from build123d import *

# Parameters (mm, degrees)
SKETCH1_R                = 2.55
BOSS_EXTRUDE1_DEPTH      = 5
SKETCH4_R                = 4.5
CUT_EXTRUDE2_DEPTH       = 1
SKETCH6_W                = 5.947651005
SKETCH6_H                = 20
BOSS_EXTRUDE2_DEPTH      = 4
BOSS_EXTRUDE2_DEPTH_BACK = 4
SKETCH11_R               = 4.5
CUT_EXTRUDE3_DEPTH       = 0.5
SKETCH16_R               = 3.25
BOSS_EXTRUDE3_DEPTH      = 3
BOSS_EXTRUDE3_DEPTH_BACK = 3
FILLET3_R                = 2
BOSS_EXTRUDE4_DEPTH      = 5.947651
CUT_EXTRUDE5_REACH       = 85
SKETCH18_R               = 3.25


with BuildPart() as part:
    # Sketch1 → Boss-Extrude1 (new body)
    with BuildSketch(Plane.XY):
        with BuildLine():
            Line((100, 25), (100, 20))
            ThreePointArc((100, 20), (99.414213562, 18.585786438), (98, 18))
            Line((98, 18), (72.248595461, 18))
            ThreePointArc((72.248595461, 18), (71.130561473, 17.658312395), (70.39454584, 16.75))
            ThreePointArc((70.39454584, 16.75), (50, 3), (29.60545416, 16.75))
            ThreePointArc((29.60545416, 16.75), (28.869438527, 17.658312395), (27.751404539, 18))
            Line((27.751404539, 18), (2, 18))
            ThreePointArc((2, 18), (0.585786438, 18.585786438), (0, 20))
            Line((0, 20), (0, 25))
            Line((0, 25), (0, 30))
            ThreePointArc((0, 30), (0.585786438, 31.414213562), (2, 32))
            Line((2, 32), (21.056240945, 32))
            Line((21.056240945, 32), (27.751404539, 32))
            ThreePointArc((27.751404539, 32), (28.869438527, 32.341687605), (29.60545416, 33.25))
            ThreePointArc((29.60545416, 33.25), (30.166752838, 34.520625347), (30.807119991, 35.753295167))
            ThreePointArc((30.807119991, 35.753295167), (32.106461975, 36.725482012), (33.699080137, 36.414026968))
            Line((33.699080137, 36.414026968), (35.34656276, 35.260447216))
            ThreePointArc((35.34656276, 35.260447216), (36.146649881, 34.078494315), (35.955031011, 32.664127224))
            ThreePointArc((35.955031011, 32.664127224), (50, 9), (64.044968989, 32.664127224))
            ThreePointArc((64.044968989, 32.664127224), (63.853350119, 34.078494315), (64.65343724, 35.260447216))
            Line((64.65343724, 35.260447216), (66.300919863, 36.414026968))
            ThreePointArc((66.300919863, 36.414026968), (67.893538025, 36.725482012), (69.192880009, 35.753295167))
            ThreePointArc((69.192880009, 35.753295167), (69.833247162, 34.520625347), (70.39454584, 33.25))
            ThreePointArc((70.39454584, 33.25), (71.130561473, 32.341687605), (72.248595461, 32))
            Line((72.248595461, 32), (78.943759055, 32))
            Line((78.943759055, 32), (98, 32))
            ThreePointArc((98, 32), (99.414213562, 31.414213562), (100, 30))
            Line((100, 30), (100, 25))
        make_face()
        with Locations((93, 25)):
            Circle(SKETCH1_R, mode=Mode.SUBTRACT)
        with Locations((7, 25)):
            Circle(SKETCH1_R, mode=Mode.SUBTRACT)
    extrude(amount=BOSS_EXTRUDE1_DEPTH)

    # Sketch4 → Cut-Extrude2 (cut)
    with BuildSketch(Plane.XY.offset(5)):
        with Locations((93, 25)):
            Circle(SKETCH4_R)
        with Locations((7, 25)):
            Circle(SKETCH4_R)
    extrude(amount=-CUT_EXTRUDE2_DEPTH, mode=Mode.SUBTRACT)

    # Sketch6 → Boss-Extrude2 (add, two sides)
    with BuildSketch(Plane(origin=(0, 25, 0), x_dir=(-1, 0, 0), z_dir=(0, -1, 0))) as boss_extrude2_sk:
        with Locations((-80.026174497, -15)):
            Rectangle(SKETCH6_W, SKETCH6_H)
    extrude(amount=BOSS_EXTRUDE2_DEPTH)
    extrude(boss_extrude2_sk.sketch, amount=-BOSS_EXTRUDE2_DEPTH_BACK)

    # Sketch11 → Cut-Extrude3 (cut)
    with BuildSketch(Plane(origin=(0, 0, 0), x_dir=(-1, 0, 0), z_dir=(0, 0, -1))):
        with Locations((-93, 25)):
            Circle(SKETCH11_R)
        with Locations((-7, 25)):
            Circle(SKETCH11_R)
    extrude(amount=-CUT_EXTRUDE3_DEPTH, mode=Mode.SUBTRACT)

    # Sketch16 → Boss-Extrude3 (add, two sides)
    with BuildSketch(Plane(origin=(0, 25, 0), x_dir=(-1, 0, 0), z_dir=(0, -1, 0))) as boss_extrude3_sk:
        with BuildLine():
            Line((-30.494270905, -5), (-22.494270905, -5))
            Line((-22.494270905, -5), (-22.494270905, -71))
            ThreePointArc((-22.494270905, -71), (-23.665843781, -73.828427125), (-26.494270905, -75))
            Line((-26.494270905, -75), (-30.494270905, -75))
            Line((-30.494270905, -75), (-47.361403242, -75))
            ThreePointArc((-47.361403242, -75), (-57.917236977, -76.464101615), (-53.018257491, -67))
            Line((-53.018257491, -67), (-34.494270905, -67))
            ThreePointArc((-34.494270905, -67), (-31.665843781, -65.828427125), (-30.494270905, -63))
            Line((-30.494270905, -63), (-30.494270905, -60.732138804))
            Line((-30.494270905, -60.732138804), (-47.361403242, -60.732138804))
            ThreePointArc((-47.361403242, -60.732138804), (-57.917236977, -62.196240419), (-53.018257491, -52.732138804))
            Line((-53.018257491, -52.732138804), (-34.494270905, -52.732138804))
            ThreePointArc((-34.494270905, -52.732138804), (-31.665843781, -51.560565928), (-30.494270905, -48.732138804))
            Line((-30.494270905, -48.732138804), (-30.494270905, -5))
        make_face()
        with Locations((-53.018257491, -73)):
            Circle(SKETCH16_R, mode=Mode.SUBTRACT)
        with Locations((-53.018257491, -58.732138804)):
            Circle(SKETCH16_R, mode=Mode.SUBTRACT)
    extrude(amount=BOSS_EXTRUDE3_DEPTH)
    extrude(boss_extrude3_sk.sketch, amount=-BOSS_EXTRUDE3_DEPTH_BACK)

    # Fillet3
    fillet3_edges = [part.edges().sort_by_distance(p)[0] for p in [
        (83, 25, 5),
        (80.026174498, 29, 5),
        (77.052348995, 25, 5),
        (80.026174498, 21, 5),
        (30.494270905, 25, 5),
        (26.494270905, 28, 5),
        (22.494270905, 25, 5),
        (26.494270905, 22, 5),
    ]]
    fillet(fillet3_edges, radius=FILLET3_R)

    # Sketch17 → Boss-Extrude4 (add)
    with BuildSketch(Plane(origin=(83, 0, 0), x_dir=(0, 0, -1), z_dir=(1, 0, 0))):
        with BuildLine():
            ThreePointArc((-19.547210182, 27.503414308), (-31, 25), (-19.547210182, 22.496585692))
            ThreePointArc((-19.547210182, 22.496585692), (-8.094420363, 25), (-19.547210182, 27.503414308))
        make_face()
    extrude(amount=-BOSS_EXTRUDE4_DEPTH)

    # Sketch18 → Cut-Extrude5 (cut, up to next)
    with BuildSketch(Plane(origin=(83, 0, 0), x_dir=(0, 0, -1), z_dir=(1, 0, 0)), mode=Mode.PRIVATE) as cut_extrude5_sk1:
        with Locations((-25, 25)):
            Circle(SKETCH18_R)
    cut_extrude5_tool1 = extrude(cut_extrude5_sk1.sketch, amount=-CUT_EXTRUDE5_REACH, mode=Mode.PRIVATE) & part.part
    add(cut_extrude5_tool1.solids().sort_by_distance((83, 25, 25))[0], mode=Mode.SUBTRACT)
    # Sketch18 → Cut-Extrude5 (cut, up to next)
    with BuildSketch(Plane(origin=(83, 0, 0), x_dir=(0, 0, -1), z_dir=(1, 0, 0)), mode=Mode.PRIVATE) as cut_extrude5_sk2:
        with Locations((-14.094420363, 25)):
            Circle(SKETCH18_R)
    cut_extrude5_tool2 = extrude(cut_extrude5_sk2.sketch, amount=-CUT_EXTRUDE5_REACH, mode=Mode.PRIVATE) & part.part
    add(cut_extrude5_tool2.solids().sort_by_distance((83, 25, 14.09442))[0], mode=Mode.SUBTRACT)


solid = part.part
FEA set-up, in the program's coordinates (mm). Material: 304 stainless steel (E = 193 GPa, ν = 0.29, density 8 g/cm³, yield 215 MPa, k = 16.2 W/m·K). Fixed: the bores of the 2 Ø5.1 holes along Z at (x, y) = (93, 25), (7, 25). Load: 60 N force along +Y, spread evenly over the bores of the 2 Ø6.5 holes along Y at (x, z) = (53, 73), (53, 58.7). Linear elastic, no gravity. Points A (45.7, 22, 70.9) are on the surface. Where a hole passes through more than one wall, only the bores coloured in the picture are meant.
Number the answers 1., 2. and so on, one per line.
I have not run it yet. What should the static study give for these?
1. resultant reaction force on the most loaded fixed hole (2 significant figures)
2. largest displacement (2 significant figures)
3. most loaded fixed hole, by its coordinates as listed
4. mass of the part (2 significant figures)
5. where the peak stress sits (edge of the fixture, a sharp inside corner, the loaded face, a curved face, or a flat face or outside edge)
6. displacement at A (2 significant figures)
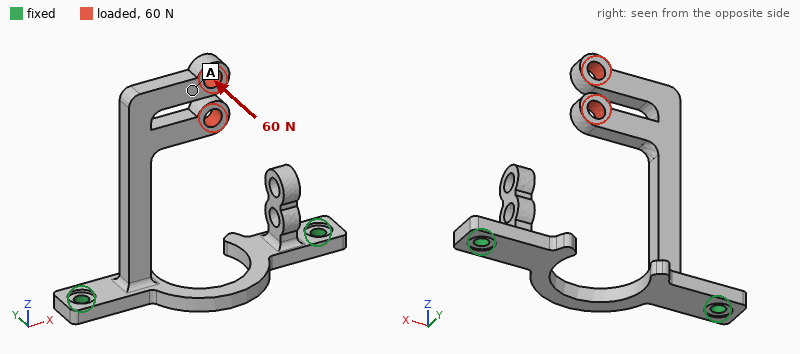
1. 55 N
2. 0.46 mm
3. (7, 25)
4. 110 g
5. a curved face
6. 0.38 mm
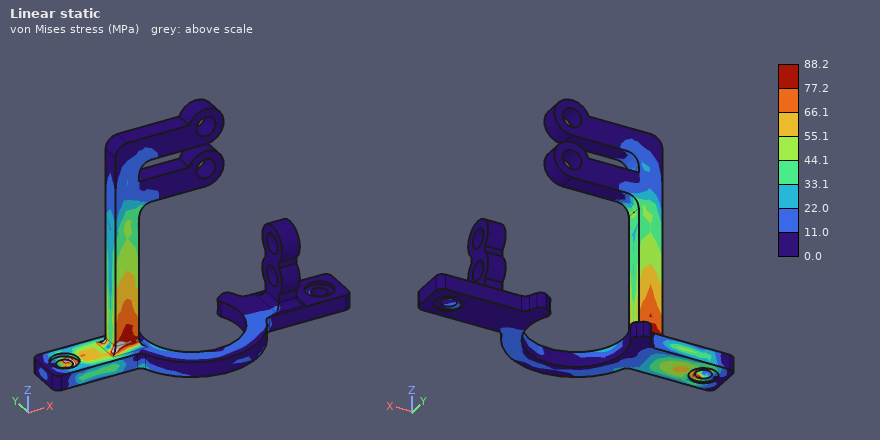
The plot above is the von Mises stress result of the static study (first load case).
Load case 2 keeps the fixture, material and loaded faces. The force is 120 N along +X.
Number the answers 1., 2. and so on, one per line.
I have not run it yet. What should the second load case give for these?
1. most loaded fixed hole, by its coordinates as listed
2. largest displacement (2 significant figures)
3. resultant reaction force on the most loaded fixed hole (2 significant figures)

1. (7, 25)
2. 0.54 mm
3. 130 N
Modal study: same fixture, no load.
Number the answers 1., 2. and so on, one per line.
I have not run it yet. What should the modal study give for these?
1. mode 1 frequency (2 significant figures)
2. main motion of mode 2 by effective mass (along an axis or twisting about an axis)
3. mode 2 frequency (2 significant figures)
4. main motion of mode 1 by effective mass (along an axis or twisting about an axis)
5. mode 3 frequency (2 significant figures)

1. 400 Hz
2. along X
3. 470 Hz
4. along Y
5. 1700 Hz
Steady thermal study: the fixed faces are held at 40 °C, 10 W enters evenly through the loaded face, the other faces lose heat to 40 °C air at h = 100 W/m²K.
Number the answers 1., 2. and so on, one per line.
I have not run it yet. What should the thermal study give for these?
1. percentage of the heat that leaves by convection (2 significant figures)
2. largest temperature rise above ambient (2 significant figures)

1. 100 %
2. 82 K
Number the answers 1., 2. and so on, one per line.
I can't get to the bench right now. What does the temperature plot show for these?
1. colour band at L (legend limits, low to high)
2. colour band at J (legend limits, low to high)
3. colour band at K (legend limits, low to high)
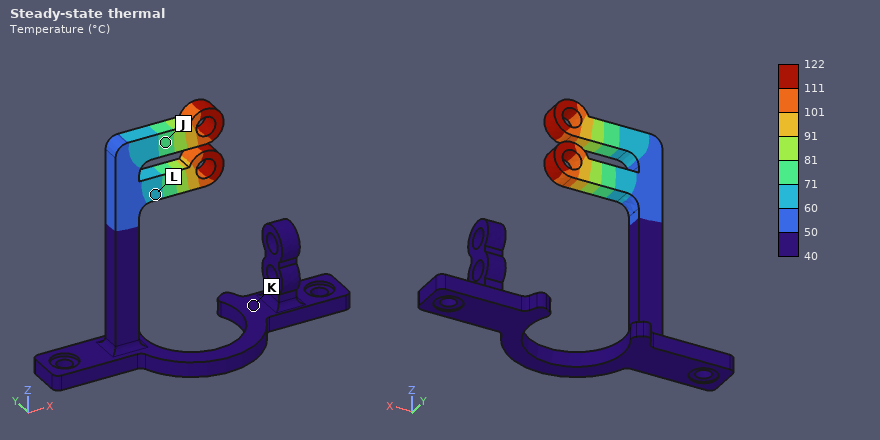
1. 60 to 71 °C
2. 71 to 81 °C
3. 40 to 50 °C
